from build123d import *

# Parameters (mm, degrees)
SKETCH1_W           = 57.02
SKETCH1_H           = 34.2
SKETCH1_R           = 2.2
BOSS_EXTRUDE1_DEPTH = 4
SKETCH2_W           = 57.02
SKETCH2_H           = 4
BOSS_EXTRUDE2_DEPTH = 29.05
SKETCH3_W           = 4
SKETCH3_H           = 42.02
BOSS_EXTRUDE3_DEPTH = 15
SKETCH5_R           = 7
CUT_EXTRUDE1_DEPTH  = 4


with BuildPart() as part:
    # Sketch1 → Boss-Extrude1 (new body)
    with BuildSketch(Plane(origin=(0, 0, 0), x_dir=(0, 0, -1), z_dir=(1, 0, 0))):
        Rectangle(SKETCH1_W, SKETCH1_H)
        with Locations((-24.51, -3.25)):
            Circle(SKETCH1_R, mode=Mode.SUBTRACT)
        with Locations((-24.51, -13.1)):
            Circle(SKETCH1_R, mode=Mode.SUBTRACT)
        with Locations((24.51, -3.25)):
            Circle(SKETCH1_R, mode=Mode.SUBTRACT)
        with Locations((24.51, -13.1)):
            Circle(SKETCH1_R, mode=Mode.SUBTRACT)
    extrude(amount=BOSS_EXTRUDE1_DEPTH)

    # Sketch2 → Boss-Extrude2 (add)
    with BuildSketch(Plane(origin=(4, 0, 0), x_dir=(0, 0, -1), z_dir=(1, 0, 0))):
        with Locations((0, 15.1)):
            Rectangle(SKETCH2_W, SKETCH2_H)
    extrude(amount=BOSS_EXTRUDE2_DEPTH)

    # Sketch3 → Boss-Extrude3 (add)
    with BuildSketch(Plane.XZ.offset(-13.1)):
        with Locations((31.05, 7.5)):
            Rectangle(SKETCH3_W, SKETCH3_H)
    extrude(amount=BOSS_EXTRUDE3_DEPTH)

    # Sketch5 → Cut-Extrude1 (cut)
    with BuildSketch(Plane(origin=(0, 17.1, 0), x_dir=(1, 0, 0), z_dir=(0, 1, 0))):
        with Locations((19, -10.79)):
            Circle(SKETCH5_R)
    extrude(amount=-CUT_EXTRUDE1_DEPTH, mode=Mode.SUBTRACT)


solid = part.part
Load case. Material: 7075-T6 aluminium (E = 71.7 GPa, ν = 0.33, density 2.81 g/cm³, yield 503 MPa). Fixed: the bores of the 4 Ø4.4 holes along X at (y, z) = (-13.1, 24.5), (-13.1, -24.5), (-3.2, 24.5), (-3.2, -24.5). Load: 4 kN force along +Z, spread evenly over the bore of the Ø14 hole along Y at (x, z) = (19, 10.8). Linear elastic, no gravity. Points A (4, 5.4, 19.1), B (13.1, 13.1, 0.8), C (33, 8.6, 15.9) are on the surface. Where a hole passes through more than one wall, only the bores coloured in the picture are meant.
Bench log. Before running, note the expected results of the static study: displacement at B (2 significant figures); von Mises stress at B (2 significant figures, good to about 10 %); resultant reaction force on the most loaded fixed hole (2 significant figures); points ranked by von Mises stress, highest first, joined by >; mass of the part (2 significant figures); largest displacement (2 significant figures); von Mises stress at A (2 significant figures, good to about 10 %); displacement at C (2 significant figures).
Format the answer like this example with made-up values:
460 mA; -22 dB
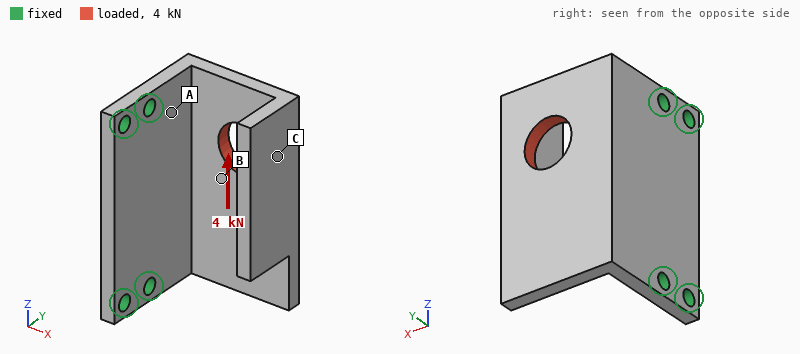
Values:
0.13 mm; 84 MPa; 2.7 kN; A > B > C; 45 g; 0.53 mm; 180 MPa; 0.40 mm
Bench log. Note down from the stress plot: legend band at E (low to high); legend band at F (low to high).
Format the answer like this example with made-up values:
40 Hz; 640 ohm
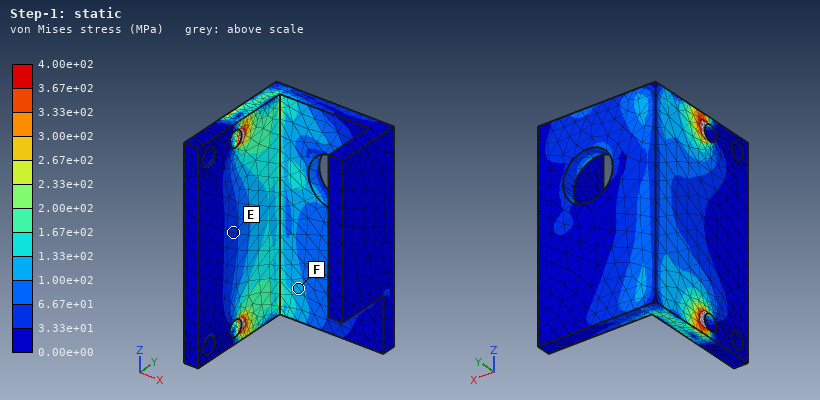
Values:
3.33e+01 to 6.67e+01 MPa; 1.00e+02 to 1.33e+02 MPa
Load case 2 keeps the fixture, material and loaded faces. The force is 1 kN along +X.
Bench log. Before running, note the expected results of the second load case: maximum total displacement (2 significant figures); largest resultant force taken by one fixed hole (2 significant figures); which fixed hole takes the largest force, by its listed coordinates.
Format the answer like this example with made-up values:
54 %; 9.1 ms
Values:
0.37 mm; 1.0 kN; (-3.2, 24.5)
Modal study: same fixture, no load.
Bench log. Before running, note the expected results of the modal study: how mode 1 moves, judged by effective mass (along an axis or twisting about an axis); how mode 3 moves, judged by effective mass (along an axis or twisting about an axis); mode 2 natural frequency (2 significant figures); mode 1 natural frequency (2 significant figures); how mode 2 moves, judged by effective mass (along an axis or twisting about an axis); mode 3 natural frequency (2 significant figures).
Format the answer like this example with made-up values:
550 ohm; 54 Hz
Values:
along Y; along X; 2400 Hz; 1200 Hz; along Z; 3200 Hz
